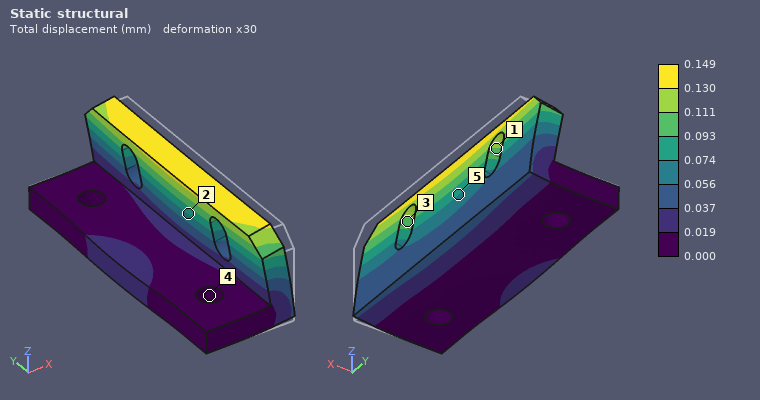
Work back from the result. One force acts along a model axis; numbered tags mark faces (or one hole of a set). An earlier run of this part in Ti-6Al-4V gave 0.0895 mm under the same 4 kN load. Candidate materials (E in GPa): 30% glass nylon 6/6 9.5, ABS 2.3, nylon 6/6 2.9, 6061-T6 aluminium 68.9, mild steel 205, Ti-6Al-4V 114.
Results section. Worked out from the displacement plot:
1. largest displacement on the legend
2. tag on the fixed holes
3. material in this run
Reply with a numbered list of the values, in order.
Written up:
1. 0.149 mm
2. 4
3. 6061-T6 aluminium
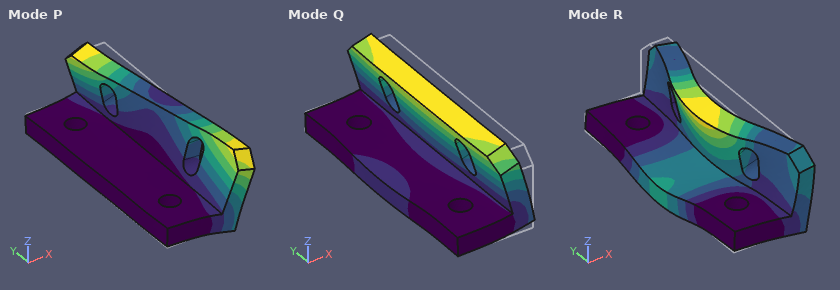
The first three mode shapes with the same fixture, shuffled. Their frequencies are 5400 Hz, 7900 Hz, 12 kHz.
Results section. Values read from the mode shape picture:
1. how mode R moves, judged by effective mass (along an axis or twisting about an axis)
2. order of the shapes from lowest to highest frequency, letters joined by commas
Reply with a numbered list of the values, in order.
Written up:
1. along Z
2. Q, P, R
